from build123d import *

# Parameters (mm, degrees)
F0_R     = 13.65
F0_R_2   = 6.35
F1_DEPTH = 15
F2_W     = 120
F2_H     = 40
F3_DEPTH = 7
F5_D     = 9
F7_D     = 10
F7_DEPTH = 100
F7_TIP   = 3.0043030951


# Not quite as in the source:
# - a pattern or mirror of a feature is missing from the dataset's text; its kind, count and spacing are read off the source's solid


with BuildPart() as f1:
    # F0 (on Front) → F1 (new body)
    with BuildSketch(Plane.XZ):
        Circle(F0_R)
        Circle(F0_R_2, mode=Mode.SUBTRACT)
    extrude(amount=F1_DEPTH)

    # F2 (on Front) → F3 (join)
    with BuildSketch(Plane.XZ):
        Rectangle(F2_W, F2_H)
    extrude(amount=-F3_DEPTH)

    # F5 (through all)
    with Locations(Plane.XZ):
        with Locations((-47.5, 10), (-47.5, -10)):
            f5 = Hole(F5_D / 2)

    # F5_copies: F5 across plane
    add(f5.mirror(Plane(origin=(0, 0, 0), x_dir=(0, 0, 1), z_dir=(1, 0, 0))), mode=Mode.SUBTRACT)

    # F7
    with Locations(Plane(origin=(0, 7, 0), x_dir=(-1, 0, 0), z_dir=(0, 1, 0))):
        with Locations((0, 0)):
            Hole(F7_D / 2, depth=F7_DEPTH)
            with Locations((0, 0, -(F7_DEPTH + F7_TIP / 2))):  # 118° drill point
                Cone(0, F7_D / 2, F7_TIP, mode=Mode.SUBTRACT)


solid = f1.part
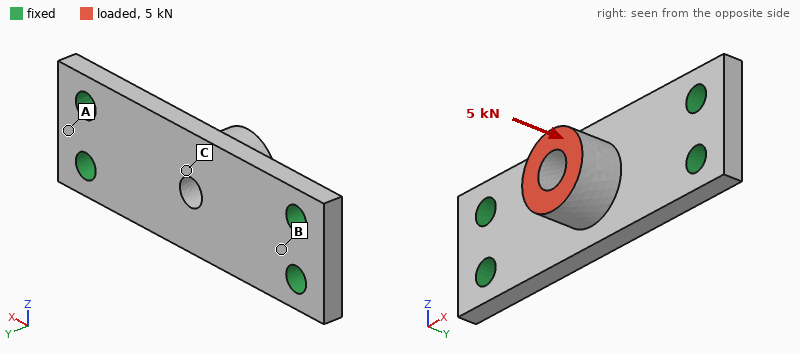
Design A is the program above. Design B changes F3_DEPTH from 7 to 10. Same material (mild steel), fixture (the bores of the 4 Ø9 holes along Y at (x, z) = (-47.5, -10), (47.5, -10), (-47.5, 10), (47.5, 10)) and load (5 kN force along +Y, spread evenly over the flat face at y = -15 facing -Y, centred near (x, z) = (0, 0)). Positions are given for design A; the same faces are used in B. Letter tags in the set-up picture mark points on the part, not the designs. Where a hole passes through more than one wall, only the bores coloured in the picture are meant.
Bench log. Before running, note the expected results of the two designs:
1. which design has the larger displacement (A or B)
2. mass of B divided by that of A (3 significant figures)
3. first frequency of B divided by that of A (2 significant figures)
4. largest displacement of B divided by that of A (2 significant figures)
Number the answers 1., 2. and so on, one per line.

1. A
2. 1.35
3. 1.4
4. 0.42
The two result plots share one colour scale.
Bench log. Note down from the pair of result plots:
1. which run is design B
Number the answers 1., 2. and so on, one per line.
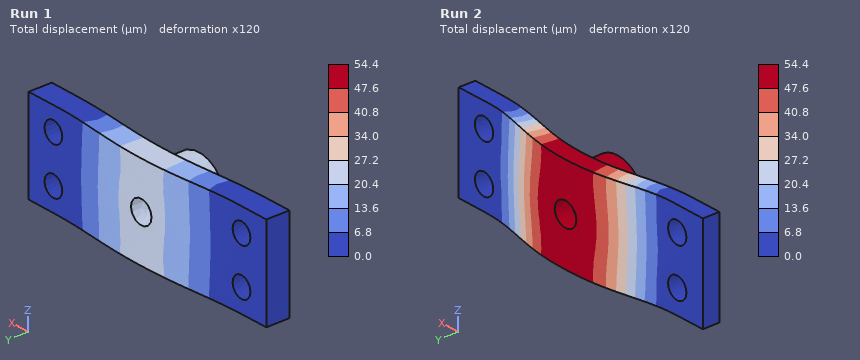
1. Run 1
